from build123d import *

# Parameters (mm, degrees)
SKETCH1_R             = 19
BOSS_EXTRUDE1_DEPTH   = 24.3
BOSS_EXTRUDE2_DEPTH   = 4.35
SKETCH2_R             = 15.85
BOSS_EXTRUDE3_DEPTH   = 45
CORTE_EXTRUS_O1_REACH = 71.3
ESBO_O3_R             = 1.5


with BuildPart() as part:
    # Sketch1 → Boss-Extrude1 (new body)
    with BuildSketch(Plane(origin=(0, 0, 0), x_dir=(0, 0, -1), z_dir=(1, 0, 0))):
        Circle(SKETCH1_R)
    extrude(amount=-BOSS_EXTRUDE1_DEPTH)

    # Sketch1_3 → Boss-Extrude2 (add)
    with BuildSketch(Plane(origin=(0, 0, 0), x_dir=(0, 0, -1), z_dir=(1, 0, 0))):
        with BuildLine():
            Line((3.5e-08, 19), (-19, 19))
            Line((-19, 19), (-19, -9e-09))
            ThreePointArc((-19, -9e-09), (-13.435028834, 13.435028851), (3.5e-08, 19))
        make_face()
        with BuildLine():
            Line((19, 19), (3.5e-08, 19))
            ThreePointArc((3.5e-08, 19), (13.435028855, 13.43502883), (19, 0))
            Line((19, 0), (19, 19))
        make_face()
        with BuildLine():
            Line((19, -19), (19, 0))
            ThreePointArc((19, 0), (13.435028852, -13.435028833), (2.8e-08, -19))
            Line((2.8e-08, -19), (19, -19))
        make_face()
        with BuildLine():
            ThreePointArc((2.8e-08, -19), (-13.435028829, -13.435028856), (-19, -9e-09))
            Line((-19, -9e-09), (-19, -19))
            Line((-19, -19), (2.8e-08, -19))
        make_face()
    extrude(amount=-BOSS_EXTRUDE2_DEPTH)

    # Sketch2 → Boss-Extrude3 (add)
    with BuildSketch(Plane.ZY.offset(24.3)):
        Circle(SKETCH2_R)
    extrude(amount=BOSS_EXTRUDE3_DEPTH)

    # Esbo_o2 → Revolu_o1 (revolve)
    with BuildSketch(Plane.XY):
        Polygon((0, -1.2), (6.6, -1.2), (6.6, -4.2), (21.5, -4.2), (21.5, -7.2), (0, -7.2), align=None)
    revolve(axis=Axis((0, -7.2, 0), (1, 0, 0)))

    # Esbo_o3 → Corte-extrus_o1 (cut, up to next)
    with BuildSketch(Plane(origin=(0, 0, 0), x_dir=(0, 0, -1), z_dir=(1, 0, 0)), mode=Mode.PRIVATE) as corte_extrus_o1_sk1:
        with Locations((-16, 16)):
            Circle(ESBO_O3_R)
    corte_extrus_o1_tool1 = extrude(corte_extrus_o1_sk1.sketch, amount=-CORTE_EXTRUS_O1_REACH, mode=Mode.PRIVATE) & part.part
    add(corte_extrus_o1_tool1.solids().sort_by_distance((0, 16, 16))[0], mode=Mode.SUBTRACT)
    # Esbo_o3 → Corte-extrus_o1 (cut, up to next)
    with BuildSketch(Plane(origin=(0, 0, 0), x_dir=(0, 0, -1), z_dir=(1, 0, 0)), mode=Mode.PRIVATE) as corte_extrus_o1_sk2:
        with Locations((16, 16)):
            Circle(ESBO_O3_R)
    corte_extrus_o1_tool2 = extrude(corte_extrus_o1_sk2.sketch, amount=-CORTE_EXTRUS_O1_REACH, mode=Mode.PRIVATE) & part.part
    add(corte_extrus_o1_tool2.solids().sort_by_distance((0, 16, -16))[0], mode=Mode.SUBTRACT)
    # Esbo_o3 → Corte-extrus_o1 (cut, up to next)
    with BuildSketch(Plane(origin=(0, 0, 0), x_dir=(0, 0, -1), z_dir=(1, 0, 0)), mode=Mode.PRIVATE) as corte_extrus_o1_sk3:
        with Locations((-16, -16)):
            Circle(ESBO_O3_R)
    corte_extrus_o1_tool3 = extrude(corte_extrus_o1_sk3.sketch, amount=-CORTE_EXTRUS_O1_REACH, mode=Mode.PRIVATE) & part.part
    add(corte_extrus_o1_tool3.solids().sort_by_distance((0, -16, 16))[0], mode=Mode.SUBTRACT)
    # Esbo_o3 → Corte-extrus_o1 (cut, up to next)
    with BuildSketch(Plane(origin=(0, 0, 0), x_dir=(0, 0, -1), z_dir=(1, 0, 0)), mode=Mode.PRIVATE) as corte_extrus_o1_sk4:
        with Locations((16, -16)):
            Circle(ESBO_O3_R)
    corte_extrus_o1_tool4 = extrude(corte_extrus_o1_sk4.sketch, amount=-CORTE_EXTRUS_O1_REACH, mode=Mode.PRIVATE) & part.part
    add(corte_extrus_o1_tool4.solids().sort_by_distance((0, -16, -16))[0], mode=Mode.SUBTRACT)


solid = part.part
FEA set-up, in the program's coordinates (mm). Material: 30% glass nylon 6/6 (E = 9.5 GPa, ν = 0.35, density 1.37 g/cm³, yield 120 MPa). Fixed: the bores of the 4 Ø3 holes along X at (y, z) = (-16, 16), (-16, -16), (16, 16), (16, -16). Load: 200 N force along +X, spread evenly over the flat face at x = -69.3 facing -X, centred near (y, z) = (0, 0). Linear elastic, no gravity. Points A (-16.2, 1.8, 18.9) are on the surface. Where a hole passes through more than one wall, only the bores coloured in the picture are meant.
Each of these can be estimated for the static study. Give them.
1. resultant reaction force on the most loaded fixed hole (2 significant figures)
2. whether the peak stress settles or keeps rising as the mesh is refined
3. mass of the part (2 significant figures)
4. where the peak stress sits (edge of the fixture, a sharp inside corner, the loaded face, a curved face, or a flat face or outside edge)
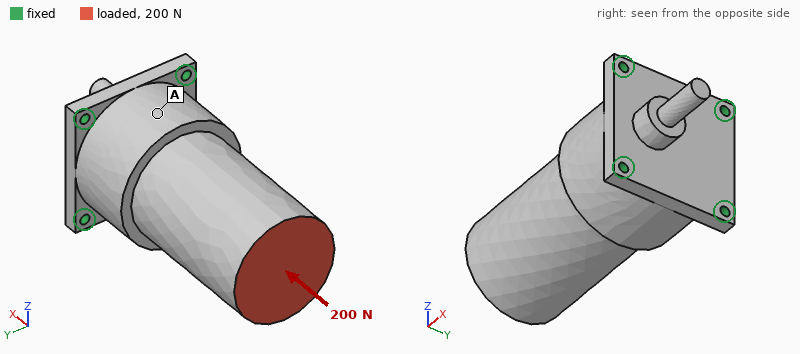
54 N
keeps rising
90 g
edge of the fixture
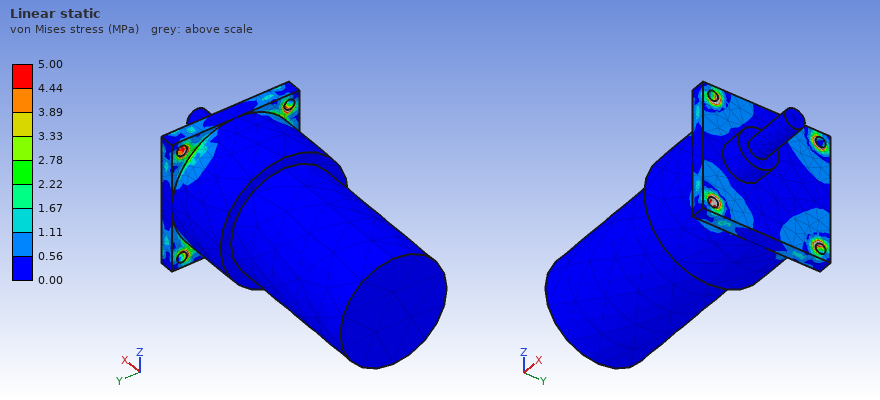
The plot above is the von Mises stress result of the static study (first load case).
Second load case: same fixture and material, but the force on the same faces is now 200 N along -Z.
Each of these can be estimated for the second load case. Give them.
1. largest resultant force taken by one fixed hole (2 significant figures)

240 N
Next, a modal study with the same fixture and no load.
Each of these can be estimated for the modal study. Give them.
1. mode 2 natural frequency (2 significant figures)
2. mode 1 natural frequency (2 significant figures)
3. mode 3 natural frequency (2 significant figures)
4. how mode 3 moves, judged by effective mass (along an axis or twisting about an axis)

1500 Hz
1500 Hz
4100 Hz
along X
